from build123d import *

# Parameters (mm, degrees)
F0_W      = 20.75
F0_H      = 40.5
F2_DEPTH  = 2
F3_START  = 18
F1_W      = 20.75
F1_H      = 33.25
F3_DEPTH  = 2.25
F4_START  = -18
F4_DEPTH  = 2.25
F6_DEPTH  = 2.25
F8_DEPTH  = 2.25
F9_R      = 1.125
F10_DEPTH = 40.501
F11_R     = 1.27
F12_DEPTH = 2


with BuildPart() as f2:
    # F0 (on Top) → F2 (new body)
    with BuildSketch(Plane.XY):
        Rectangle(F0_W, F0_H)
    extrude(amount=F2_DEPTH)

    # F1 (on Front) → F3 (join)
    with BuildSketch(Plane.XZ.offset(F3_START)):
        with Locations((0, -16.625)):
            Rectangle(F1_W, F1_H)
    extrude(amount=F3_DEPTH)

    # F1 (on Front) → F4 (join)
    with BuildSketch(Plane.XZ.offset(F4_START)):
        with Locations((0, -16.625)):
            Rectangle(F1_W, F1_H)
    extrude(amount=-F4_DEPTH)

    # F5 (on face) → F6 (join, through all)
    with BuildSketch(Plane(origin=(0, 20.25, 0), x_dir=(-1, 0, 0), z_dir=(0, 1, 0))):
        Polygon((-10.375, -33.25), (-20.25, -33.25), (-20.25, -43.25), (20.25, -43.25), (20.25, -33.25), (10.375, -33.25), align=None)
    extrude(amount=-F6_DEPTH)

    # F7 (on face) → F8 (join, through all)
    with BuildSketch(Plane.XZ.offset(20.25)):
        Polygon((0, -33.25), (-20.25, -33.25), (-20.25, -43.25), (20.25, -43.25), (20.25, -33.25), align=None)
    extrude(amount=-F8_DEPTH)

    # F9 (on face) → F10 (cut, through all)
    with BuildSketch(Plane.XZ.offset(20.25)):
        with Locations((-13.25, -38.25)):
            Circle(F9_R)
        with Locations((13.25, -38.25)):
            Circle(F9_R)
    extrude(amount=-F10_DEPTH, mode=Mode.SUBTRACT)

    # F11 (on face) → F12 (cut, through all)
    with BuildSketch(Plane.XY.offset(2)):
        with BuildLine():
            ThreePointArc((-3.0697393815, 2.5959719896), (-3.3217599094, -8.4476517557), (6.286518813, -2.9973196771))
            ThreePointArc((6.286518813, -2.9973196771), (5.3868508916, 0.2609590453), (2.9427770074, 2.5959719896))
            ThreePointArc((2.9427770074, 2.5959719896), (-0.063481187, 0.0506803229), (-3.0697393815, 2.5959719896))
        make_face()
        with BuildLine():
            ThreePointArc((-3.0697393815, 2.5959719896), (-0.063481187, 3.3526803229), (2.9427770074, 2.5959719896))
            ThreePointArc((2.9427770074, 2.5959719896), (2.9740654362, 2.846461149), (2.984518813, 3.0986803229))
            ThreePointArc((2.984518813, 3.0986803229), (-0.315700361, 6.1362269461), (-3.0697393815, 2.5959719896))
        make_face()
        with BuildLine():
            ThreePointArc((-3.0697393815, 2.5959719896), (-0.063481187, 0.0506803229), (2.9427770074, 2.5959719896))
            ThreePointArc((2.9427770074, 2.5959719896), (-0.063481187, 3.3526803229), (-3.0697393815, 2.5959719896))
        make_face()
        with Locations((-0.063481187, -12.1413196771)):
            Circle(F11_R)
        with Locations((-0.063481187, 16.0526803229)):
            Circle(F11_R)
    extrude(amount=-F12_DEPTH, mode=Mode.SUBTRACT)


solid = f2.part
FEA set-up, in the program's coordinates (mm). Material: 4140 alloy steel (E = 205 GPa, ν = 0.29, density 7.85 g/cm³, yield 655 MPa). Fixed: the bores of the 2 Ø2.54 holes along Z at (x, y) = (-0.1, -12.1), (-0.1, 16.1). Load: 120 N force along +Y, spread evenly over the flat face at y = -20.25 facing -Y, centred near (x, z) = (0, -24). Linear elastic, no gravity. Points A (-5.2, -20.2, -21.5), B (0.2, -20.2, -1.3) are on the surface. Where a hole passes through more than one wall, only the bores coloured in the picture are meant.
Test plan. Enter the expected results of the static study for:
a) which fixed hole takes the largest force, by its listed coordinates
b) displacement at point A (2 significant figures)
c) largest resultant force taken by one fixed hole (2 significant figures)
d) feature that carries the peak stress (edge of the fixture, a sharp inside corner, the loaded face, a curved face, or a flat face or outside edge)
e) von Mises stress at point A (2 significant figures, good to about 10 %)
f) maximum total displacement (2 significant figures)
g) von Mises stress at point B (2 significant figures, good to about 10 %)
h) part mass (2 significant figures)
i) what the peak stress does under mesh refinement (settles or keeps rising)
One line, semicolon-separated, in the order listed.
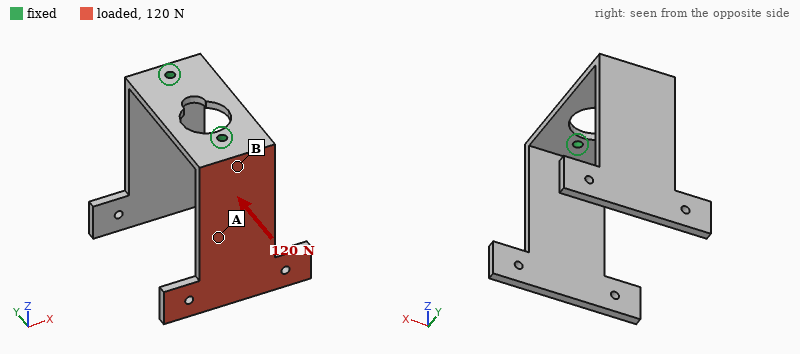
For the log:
(-0.1, -12.1); 0.30 mm; 120 N; edge of the fixture; 49 MPa; 0.70 mm; 140 MPa; 49 g; keeps rising
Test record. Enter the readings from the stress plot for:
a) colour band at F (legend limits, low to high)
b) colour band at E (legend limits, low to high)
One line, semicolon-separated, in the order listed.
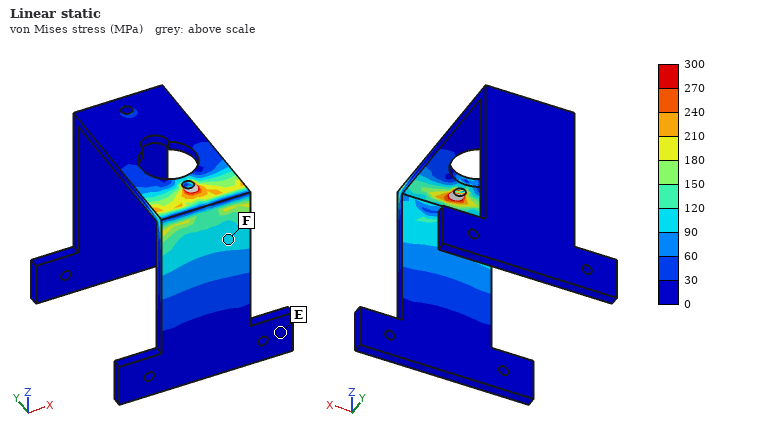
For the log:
90 to 120 MPa; 0 to 30 MPa
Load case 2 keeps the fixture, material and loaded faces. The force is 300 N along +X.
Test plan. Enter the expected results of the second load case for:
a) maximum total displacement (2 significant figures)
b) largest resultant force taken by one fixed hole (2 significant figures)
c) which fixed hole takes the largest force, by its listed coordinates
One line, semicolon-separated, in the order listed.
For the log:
0.56 mm; 360 N; (-0.1, -12.1)
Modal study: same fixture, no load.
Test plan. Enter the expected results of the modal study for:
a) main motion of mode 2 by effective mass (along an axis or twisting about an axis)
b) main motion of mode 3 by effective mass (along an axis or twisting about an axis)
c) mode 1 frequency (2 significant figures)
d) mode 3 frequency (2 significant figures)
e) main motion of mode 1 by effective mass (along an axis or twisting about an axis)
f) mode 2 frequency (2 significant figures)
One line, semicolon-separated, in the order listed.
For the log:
along Y; along X; 550 Hz; 970 Hz; along Y; 650 Hz
